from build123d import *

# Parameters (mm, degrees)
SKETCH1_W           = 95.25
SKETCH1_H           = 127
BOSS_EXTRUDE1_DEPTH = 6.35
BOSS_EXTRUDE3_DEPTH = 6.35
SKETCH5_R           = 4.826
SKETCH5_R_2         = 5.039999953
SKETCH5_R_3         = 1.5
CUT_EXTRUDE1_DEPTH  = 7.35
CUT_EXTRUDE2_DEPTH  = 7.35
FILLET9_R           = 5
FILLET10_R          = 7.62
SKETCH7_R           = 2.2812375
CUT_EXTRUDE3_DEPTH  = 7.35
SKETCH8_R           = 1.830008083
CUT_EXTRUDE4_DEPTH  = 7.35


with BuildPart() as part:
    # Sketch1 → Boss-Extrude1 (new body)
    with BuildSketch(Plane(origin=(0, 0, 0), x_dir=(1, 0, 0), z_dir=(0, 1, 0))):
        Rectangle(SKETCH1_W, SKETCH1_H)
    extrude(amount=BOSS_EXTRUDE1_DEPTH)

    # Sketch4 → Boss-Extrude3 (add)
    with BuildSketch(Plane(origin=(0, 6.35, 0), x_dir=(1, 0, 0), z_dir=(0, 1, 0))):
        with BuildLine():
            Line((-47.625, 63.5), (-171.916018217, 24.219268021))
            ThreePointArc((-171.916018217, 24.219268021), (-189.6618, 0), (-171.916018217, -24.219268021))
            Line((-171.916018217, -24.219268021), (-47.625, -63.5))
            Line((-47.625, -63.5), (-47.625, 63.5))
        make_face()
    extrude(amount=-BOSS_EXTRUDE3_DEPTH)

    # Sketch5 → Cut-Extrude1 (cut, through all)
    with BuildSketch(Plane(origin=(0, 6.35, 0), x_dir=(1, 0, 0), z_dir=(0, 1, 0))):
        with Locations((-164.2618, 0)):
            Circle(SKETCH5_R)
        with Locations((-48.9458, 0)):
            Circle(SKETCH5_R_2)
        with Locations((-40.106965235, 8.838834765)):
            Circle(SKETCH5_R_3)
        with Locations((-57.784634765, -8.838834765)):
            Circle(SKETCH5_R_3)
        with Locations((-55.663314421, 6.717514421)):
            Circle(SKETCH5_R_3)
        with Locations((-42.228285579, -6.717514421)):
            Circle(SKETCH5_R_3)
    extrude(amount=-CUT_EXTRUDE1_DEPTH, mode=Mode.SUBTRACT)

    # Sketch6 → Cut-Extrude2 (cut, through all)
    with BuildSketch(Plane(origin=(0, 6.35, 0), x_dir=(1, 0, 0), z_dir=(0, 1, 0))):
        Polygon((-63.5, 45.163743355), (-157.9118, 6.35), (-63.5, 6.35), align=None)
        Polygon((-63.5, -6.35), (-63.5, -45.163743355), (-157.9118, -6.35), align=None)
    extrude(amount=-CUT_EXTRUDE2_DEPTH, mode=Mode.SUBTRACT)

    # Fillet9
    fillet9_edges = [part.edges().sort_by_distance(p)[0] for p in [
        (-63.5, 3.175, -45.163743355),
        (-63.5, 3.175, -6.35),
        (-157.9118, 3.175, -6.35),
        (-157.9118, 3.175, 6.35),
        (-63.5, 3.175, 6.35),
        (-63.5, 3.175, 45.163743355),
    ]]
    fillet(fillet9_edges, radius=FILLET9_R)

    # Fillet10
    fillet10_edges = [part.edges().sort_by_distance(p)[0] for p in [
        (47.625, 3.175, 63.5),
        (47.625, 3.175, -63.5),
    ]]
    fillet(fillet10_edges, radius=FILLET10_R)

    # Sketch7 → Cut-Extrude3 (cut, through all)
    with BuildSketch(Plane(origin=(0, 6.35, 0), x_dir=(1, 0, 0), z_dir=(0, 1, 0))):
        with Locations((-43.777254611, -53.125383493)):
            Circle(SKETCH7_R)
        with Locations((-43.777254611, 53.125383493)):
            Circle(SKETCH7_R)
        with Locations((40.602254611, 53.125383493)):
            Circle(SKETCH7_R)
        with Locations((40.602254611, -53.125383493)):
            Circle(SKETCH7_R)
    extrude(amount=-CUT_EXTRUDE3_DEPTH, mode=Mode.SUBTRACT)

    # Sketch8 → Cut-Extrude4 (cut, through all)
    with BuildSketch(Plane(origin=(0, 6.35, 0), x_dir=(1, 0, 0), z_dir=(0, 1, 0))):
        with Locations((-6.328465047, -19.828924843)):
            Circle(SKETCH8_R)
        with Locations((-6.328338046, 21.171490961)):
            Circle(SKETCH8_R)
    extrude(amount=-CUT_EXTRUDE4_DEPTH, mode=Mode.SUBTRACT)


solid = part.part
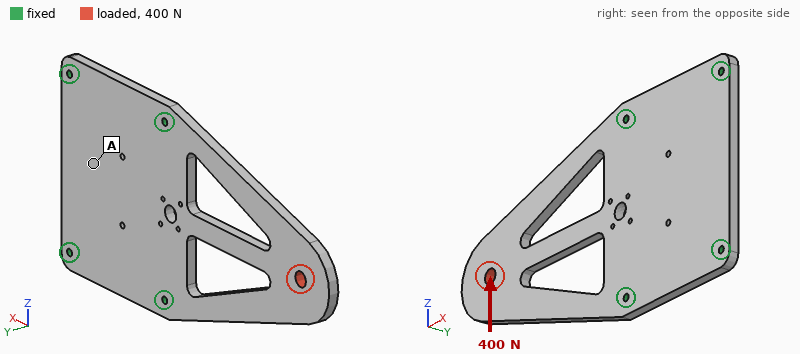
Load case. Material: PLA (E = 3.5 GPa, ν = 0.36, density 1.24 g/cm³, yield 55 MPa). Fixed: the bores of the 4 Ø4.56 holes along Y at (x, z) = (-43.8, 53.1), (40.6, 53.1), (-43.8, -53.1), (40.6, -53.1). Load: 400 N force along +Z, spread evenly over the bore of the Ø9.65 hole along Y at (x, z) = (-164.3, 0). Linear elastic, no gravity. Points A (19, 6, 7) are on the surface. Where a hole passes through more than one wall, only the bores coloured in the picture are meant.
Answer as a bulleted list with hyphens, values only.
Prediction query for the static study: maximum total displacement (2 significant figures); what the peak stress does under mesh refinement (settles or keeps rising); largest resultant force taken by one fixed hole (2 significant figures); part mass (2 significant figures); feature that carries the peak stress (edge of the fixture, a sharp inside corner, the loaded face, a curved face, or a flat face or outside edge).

- 0.47 mm
- keeps rising
- 470 N
- 160 g
- a sharp inside corner
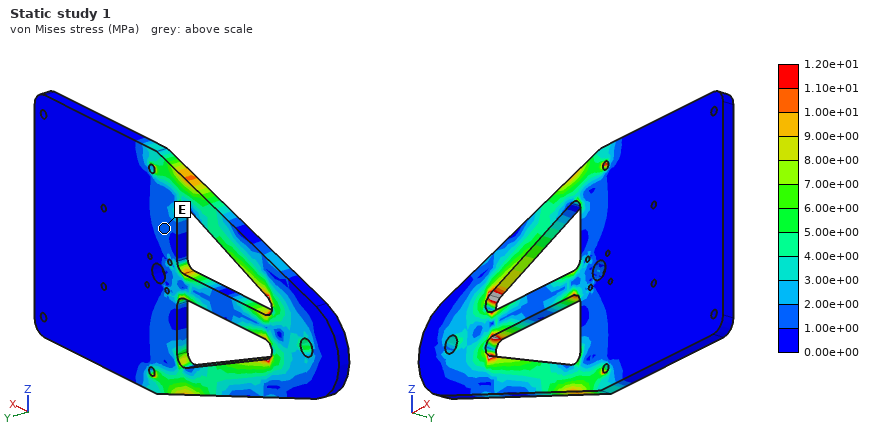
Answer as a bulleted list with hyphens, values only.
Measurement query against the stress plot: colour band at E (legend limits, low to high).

- 1.00e+00 to 2.00e+00 MPa
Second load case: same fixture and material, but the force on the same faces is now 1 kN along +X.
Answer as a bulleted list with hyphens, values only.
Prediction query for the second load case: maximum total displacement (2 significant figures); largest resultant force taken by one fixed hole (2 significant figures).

- 0.16 mm
- 420 N
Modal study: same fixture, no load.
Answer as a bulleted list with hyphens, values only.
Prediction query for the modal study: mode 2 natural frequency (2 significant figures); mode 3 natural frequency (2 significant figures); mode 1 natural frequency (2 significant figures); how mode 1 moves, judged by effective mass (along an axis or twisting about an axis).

- 390 Hz
- 510 Hz
- 83 Hz
- along Y
